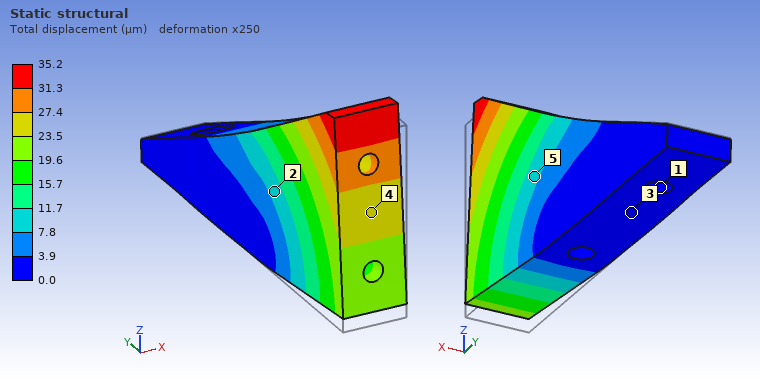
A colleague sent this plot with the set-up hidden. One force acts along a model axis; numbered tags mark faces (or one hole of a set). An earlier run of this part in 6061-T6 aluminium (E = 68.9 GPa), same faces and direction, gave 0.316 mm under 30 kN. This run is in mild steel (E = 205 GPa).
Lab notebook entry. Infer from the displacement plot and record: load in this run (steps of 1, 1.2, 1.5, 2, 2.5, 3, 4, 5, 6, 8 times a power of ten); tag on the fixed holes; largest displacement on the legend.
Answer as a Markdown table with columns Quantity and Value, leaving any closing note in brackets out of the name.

| Quantity | Value |
|---|---|
| load in this run | 10 kN |
| tag on the fixed holes | 1 |
| largest displacement on the legend | 35.2 µm |
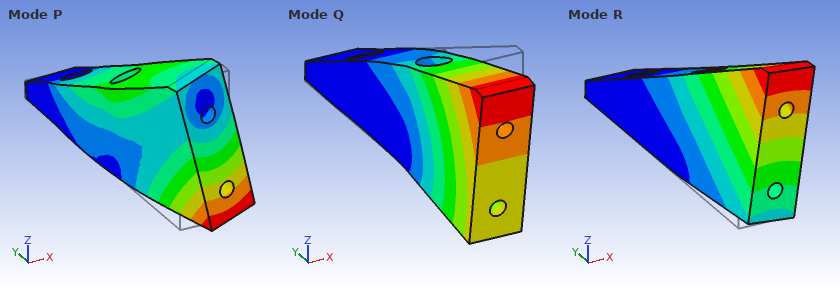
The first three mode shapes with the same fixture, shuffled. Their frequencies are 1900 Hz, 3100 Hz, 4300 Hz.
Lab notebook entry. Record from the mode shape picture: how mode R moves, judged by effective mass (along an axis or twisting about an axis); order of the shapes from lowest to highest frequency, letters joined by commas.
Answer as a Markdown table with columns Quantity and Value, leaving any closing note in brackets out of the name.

| Quantity | Value |
|---|---|
| how mode R moves, judged by effective mass | along X |
| order of the shapes from lowest to highest frequency, letters joined by commas | R, Q, P |
